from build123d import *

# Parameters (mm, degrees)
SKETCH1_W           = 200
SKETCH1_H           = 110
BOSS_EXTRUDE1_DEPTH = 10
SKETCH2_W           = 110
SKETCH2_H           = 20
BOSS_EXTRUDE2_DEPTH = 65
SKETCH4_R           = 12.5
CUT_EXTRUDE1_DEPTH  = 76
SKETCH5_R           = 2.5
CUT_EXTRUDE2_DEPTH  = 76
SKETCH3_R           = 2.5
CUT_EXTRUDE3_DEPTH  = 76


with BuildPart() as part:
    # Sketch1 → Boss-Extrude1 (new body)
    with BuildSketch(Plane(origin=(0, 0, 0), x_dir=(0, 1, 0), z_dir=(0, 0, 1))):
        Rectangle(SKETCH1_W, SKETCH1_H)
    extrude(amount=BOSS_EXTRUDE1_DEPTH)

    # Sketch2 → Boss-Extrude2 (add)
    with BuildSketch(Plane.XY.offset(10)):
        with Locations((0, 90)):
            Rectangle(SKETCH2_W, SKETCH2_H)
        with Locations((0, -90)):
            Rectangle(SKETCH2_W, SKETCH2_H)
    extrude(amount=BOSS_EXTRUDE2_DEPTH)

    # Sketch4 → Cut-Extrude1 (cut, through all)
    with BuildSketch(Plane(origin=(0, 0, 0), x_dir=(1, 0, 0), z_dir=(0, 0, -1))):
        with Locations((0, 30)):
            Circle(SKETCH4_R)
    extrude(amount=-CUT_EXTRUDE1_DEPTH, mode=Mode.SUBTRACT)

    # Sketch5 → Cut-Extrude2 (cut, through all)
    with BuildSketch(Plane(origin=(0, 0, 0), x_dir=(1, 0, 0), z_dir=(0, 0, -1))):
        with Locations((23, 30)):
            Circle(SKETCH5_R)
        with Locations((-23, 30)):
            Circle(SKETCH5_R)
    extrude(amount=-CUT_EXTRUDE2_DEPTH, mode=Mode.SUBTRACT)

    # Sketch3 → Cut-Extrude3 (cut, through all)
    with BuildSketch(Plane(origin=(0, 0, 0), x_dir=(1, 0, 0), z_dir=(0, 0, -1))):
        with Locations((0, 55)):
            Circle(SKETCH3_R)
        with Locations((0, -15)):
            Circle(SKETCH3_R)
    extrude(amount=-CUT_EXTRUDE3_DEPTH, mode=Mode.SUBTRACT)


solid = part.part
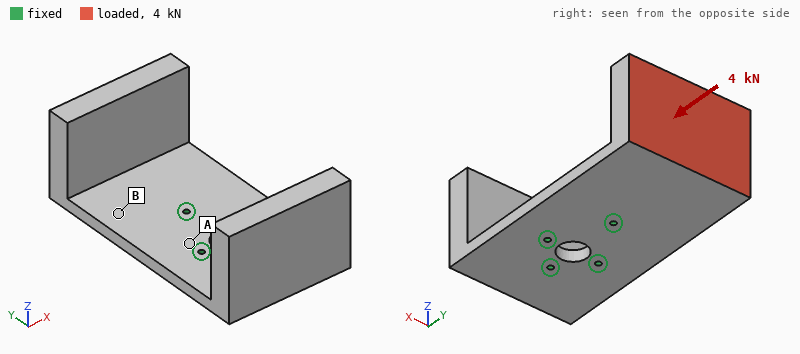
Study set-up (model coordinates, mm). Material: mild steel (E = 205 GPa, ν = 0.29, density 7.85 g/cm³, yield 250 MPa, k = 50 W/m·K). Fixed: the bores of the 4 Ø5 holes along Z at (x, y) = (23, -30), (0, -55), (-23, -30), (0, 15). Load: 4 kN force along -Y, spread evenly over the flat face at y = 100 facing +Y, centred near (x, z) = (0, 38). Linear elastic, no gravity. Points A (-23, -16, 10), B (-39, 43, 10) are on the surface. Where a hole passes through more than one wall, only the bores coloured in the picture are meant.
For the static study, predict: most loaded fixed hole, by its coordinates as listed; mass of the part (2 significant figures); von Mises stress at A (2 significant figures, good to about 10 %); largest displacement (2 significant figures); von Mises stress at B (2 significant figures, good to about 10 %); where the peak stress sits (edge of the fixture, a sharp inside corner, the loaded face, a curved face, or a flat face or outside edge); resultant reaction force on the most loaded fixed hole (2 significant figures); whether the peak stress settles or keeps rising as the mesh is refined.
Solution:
(0, 15)
3.9 kg
11 MPa
0.46 mm
70 MPa
edge of the fixture
3.0 kN
keeps rising
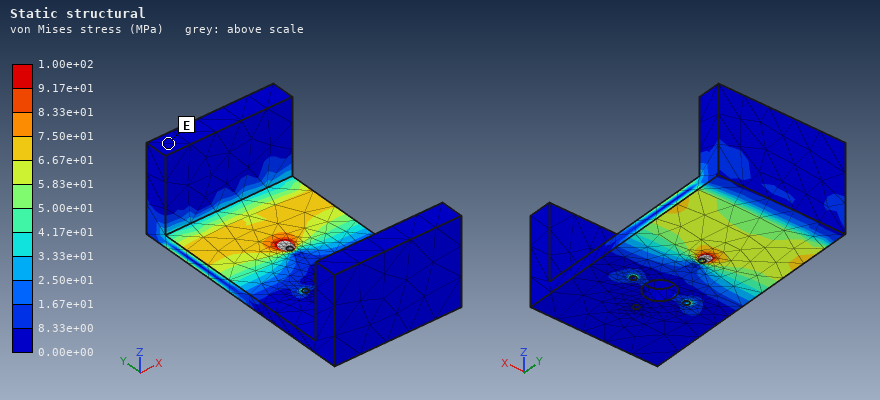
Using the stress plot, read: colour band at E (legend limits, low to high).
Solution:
0.00e+00 to 8.33e+00 MPa
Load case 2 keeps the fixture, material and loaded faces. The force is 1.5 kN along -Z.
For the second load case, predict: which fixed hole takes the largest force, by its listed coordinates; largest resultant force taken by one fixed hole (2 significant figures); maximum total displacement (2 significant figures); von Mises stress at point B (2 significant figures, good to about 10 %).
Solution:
(0, 15)
3.4 kN
0.31 mm
43 MPa
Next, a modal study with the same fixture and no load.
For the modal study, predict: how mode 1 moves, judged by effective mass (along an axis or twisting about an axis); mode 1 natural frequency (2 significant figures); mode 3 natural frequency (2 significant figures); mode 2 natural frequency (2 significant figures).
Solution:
along Z
350 Hz
670 Hz
550 Hz
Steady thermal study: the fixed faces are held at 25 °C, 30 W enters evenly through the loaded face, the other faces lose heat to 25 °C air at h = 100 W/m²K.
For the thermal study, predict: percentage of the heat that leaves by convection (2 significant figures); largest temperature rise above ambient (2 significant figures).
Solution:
89 %
14 K
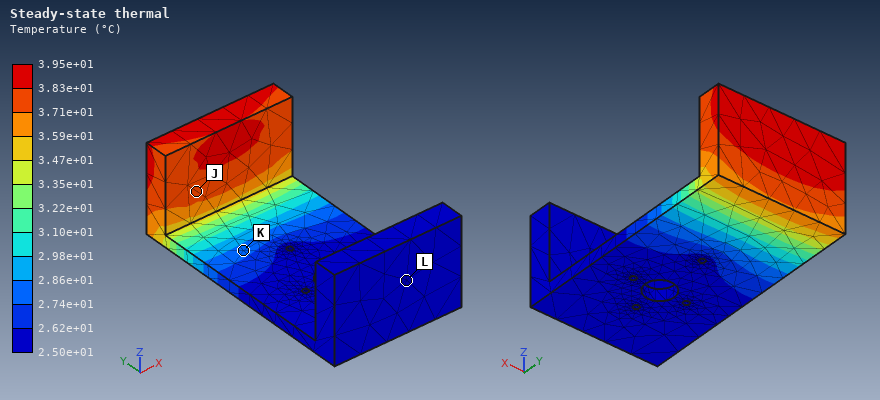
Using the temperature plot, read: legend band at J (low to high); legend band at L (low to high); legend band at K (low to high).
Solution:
3.71e+01 to 3.83e+01 °C
2.50e+01 to 2.62e+01 °C
2.74e+01 to 2.86e+01 °C
